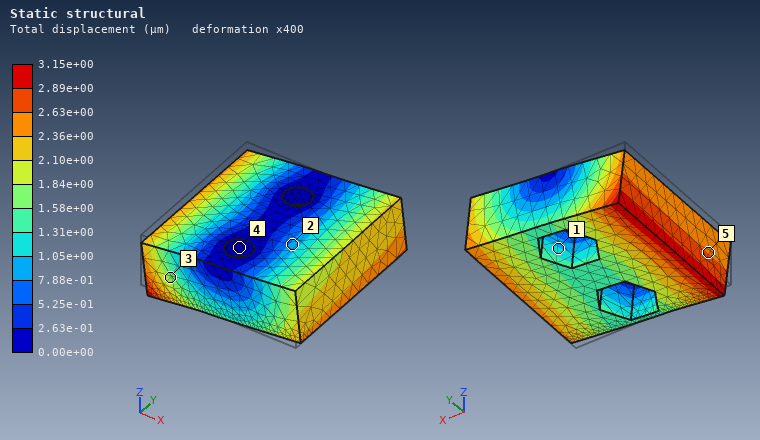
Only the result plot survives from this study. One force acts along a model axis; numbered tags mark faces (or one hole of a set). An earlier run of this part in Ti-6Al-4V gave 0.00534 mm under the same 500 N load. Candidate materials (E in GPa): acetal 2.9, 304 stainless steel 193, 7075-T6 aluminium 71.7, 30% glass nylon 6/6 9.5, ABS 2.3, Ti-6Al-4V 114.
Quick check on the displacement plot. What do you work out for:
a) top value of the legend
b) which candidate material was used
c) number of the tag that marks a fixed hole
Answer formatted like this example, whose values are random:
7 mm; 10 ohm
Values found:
3.15e+00 µm; 304 stainless steel; 4
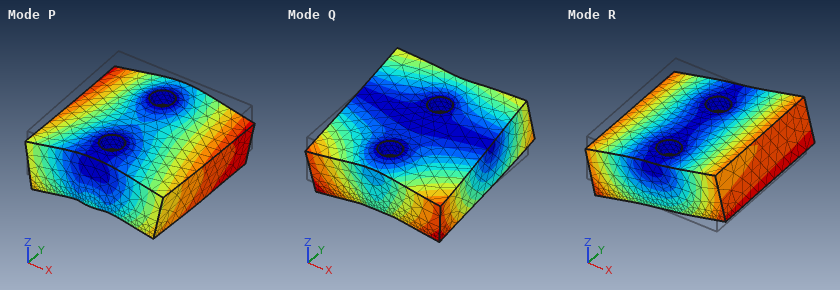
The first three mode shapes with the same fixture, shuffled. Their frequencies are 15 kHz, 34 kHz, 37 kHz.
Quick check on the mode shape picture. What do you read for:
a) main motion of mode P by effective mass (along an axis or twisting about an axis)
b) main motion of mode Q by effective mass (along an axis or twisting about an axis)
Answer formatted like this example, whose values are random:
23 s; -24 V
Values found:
along Z; along Y
